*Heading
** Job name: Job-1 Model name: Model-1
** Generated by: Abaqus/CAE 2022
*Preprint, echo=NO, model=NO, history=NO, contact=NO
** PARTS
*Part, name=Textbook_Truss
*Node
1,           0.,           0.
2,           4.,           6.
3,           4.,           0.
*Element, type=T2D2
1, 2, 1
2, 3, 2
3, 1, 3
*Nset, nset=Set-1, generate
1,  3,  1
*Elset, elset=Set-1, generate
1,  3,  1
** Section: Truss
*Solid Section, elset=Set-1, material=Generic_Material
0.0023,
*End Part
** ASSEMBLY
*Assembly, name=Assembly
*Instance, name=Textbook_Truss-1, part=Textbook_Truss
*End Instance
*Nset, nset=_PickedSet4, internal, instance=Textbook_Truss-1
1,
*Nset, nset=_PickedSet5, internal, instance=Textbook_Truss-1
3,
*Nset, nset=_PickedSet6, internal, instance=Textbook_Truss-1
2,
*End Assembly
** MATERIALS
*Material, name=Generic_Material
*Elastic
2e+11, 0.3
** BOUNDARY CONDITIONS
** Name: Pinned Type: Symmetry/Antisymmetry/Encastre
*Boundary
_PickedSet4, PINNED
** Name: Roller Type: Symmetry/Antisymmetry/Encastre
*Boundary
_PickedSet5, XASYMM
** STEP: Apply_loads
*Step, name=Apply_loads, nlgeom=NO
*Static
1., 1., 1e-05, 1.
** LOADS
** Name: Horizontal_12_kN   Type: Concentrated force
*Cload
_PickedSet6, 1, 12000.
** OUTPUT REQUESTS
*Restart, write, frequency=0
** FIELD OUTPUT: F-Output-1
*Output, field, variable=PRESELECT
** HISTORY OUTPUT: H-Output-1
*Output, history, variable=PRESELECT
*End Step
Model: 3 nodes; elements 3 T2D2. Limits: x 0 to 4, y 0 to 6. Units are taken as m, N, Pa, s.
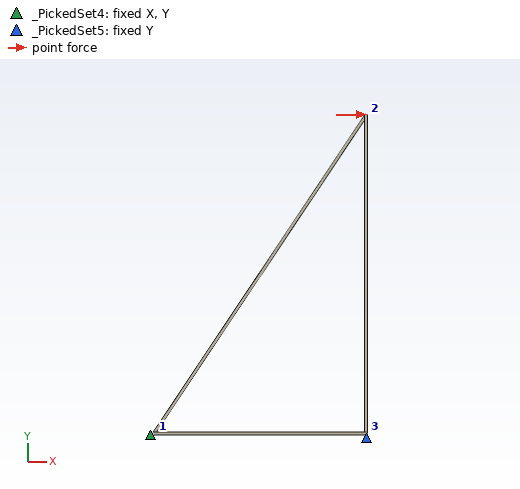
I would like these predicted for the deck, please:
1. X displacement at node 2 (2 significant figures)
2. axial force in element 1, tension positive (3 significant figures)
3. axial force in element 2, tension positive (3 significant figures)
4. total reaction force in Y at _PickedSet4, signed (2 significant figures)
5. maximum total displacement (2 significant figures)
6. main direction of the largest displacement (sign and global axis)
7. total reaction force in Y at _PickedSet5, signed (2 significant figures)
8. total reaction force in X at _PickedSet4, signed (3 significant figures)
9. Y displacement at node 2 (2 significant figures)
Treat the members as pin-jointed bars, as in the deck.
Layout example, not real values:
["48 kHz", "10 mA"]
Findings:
["9.6e-04 m", "21600 N", "-18000 N", "-18000 N", "9.9e-04 m", "+X", "18000 N", "-12000 N", "-2.3e-04 m"]
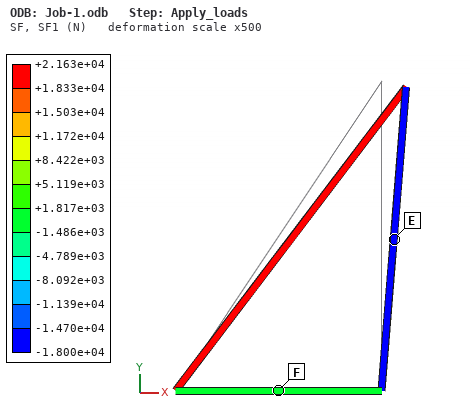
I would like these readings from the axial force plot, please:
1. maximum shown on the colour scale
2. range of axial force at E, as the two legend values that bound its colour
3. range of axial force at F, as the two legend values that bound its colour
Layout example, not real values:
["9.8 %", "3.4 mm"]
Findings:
["+2.163e+04 N", "-1.800e+04 to -1.470e+04 N", "-1.486e+03 to +1.817e+03 N"]
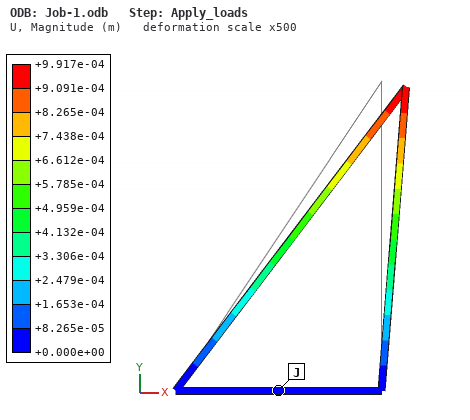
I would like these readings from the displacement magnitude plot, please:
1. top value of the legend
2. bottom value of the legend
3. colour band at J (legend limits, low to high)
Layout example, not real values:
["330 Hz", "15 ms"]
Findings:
["+9.917e-04 m", "+0.000e+00 m", "+0.000e+00 to +8.265e-05 m"]
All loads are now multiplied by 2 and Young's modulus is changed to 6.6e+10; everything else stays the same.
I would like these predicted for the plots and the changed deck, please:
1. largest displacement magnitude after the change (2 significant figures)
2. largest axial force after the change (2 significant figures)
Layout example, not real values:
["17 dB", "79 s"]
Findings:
["0.0060 m", "43000 N"]
